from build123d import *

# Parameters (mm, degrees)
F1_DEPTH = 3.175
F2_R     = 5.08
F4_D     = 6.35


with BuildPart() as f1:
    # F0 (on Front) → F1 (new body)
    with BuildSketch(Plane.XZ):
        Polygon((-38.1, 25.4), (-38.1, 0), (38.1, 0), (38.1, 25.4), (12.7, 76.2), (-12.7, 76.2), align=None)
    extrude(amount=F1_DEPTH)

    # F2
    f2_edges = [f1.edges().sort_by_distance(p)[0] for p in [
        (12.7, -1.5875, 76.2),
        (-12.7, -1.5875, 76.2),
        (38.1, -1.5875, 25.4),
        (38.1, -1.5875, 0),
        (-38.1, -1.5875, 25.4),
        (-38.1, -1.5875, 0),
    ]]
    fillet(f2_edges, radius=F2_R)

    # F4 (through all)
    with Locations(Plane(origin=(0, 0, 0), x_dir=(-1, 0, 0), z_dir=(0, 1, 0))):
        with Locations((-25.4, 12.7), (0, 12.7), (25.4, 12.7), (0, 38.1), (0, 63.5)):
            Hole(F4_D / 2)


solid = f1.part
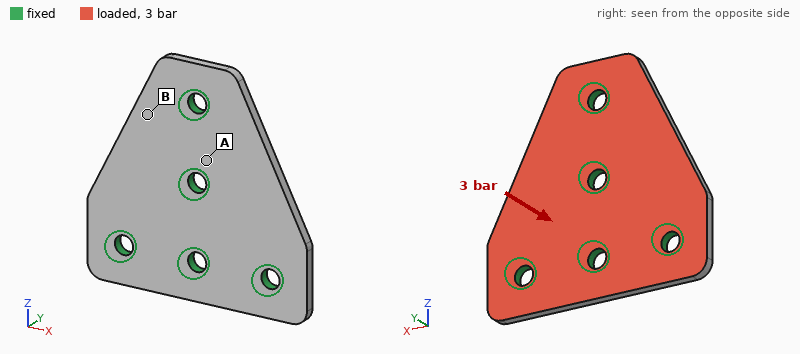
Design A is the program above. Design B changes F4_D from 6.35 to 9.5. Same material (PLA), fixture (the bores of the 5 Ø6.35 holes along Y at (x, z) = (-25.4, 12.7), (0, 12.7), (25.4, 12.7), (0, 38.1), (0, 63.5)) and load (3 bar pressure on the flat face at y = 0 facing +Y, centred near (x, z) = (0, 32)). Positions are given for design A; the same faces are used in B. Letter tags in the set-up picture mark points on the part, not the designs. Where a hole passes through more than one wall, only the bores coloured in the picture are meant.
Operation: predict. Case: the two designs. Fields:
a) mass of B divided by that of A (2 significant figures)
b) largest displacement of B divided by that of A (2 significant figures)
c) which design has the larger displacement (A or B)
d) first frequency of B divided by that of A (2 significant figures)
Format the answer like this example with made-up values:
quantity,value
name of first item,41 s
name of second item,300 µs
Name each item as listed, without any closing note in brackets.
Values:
quantity,value
mass of B divided by that of A,0.95
largest displacement of B divided by that of A,0.78
which design has the larger displacement,A
first frequency of B divided by that of A,1.2
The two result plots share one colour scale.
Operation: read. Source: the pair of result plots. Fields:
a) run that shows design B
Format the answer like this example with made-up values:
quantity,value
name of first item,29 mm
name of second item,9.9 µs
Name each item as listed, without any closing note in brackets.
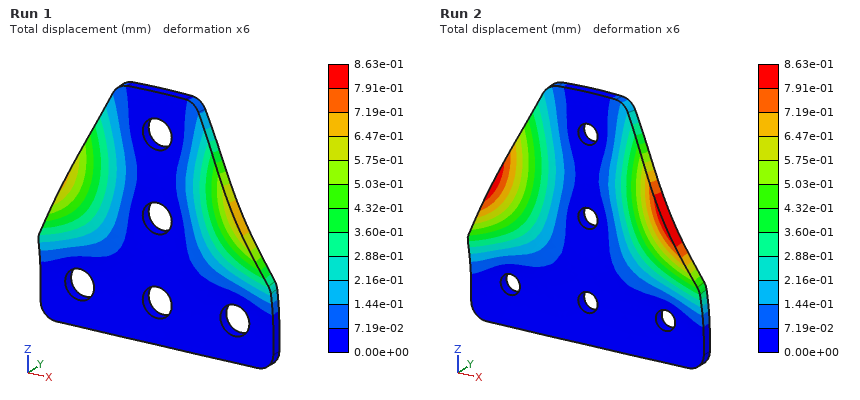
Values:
quantity,value
run that shows design B,Run 1
